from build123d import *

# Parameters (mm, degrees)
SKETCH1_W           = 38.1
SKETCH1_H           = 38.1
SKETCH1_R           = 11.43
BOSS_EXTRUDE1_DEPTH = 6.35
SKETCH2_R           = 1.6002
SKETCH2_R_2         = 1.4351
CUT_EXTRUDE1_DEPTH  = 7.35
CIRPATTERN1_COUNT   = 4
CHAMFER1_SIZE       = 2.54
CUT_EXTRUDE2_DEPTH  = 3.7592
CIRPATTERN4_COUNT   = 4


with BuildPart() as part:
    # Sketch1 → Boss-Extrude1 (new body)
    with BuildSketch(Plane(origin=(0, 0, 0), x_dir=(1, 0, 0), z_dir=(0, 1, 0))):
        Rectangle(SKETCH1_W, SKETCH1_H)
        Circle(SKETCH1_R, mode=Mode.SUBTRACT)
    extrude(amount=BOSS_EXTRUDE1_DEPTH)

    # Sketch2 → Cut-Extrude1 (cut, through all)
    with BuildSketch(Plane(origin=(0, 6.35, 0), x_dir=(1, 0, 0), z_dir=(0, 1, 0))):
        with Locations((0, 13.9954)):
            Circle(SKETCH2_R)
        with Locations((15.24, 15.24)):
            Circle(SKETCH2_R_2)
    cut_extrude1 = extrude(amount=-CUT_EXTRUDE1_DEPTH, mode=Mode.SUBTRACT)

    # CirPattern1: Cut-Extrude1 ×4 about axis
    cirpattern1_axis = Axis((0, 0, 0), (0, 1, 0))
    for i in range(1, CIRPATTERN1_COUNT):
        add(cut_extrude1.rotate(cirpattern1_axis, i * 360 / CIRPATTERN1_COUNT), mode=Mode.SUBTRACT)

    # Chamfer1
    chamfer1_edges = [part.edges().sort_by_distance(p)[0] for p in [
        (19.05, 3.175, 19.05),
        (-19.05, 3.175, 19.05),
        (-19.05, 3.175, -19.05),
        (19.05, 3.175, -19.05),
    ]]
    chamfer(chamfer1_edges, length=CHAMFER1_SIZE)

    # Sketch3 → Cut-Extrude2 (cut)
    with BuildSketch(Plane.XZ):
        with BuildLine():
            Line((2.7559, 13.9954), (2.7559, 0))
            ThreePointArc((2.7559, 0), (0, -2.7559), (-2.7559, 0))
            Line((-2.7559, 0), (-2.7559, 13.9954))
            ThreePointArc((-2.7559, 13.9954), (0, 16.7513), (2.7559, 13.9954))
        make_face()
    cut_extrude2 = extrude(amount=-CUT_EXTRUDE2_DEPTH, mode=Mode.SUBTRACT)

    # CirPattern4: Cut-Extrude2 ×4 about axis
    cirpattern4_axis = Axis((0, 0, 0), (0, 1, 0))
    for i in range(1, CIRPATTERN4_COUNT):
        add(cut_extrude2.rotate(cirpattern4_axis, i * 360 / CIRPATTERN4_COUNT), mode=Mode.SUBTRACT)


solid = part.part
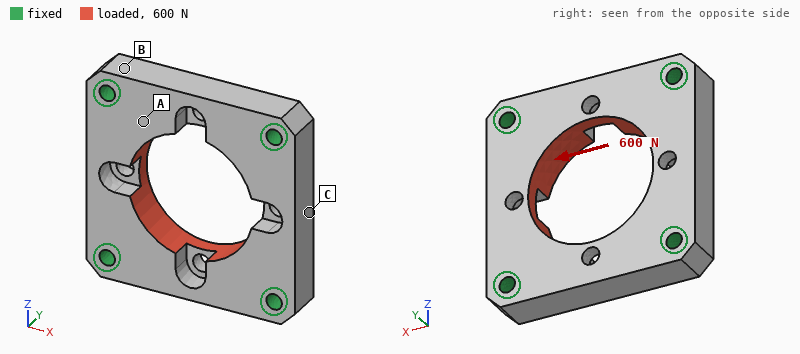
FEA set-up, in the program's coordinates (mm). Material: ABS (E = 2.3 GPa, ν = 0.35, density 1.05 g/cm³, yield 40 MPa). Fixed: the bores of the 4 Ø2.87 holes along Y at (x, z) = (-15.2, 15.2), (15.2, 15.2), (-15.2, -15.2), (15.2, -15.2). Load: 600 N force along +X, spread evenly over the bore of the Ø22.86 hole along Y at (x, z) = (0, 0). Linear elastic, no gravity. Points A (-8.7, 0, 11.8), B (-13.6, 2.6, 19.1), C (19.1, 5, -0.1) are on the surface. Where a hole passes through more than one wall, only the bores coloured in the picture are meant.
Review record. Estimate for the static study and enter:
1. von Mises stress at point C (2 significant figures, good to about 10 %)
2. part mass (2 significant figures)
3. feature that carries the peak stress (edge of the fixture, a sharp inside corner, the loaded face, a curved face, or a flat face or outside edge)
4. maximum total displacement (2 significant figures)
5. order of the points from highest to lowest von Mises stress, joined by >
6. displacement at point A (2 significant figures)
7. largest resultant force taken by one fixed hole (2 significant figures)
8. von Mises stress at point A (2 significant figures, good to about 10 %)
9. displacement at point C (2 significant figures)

4.2 MPa
6.2 g
a curved face
52 µm
C > A > B
19 µm
150 N
2.2 MPa
41 µm
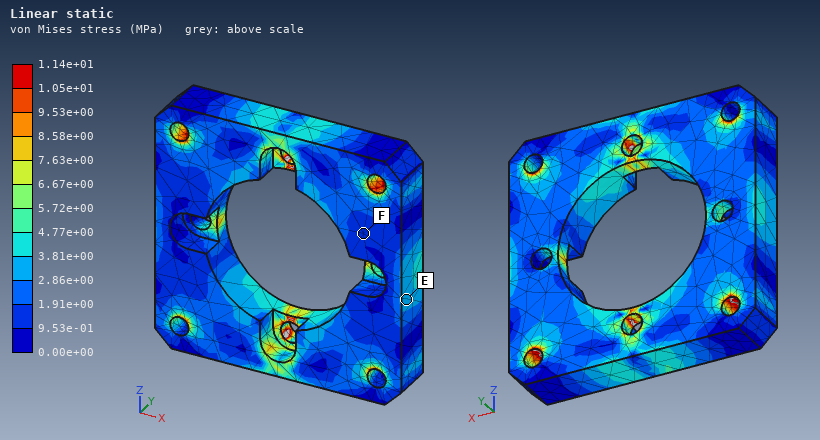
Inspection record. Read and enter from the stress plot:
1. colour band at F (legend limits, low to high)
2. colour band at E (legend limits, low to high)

9.53e-01 to 1.91e+00 MPa
2.86e+00 to 3.81e+00 MPa
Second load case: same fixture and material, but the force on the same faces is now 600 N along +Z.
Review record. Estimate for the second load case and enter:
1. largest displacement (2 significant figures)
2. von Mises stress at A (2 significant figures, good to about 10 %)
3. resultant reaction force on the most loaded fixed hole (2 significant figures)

52 µm
1.8 MPa
150 N
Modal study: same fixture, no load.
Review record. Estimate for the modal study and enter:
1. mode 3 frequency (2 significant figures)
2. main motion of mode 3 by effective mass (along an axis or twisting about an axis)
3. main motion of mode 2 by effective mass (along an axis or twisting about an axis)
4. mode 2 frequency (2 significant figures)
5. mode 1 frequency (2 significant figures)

8600 Hz
twisting about Z
along Y
8100 Hz
6800 Hz
